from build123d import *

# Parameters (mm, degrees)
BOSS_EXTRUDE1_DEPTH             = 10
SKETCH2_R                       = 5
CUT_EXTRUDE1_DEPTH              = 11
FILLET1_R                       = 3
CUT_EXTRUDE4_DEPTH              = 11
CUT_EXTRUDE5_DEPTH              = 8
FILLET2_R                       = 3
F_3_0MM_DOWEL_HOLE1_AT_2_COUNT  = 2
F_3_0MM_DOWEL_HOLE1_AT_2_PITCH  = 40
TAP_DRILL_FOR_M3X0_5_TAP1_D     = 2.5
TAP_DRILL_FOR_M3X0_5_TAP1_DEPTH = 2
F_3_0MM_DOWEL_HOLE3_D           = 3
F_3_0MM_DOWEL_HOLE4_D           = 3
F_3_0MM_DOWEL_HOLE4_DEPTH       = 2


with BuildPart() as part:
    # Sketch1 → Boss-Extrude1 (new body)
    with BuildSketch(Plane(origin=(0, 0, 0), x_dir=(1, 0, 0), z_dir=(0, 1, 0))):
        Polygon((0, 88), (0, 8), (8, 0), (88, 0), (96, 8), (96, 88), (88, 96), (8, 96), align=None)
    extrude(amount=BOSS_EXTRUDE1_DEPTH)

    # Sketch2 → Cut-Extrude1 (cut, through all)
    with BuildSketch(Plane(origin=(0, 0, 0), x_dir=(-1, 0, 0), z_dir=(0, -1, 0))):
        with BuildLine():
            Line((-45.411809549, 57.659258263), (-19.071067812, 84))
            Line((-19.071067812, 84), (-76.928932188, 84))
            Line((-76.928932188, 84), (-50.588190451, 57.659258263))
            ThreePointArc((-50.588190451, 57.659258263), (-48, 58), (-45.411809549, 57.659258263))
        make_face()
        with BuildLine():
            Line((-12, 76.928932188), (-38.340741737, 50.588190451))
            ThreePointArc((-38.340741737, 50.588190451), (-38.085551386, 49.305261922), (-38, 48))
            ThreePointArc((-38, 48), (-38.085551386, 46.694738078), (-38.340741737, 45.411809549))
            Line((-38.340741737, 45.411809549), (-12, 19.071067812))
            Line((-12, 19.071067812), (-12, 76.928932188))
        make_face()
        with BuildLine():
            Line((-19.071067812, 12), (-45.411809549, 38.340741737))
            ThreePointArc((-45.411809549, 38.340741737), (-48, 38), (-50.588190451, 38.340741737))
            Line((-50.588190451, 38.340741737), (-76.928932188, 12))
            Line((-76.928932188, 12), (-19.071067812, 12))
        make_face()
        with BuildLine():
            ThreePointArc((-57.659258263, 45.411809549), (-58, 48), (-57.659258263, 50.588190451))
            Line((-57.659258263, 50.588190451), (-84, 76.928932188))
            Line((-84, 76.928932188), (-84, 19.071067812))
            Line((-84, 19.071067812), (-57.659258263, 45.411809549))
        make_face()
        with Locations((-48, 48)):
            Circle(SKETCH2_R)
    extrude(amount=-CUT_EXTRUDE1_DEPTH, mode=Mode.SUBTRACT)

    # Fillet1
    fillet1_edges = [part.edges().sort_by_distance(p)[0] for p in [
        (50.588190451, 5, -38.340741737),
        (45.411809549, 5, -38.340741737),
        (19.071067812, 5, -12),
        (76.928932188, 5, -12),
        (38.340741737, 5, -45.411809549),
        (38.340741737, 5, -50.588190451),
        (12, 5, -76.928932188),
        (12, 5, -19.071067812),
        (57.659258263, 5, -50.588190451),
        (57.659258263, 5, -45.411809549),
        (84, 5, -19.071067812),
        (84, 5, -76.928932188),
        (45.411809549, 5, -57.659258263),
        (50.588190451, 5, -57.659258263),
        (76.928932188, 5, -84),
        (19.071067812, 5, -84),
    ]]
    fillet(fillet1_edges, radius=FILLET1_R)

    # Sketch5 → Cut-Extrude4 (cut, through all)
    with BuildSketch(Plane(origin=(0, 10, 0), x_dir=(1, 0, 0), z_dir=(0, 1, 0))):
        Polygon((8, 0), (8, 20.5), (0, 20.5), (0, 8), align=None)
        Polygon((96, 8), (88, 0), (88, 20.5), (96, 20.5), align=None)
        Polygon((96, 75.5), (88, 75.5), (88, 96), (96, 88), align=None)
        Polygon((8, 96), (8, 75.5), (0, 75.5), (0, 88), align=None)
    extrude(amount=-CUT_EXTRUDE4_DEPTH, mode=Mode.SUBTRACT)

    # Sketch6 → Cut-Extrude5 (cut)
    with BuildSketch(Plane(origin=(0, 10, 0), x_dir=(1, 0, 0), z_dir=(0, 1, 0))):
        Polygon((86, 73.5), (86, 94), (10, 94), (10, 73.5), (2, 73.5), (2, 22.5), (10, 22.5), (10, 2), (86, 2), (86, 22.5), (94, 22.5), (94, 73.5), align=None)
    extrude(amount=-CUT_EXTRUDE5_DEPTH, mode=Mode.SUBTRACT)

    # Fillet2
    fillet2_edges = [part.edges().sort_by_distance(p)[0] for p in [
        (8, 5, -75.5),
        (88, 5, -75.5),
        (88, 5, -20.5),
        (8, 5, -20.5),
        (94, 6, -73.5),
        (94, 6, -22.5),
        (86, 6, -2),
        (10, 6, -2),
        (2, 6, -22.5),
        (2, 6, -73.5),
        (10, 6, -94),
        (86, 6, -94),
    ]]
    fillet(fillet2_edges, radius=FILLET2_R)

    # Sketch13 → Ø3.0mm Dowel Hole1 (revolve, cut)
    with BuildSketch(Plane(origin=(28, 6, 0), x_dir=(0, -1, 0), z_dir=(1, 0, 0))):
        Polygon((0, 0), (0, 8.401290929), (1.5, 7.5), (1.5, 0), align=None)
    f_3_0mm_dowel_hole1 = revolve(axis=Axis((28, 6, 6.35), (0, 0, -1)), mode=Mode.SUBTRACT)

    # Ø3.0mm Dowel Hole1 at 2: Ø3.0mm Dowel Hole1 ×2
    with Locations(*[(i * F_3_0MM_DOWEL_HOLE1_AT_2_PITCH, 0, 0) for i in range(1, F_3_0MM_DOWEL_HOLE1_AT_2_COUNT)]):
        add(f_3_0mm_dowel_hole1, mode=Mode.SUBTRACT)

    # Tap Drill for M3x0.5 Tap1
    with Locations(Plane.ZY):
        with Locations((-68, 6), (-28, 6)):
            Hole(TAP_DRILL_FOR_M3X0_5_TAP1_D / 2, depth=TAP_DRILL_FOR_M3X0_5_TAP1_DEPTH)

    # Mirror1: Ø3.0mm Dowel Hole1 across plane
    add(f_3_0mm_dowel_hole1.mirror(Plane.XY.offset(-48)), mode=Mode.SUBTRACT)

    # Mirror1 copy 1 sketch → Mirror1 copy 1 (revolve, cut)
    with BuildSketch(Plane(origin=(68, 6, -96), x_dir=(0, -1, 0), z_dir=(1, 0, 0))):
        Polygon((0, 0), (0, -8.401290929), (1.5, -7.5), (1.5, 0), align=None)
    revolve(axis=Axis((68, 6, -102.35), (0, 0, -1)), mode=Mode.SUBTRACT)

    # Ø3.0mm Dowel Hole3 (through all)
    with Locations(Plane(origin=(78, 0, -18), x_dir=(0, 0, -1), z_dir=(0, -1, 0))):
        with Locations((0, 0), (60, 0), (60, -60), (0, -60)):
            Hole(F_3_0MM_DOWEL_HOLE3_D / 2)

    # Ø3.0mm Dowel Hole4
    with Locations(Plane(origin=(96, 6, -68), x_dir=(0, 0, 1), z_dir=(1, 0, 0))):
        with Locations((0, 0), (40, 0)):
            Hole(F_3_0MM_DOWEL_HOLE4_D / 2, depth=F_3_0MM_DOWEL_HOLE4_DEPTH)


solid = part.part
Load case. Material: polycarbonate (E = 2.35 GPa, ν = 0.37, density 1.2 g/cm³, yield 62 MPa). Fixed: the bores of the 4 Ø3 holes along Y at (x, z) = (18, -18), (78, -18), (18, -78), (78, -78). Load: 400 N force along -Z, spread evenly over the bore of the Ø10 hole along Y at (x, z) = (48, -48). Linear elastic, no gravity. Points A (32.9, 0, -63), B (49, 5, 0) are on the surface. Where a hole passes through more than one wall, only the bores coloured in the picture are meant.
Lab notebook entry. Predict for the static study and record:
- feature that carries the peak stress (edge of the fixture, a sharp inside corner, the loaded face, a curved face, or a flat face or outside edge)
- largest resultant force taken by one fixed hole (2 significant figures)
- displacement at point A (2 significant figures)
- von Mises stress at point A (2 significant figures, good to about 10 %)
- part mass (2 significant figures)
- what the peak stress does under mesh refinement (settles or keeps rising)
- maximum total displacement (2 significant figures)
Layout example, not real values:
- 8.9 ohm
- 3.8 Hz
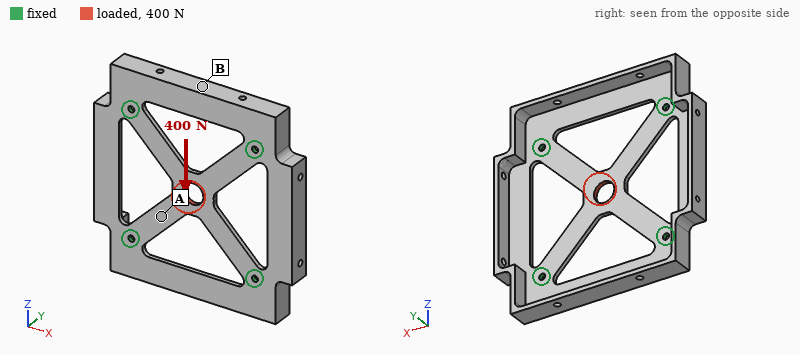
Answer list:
- edge of the fixture
- 130 N
- 0.086 mm
- 6.8 MPa
- 20 g
- keeps rising
- 0.18 mm
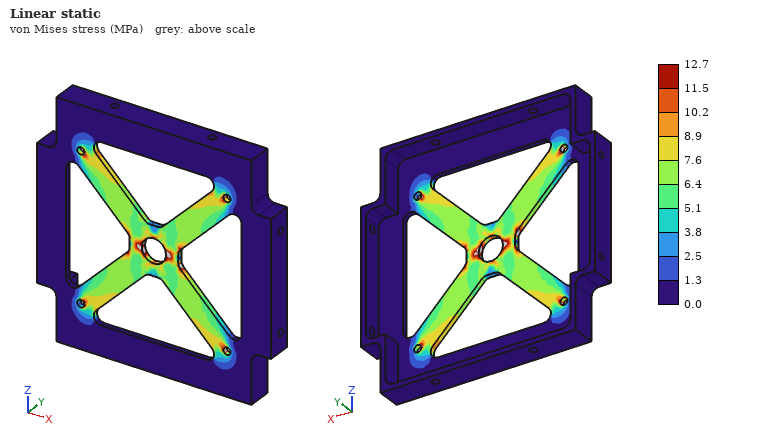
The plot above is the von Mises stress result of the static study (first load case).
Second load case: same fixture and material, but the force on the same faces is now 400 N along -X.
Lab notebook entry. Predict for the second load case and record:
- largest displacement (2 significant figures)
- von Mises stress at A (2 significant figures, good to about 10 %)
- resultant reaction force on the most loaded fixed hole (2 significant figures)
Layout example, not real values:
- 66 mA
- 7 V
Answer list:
- 0.18 mm
- 6.9 MPa
- 130 N
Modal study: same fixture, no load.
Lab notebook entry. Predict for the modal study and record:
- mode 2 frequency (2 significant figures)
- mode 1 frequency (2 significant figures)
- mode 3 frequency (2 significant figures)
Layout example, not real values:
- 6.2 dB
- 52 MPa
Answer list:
- 640 Hz
- 490 Hz
- 700 Hz
